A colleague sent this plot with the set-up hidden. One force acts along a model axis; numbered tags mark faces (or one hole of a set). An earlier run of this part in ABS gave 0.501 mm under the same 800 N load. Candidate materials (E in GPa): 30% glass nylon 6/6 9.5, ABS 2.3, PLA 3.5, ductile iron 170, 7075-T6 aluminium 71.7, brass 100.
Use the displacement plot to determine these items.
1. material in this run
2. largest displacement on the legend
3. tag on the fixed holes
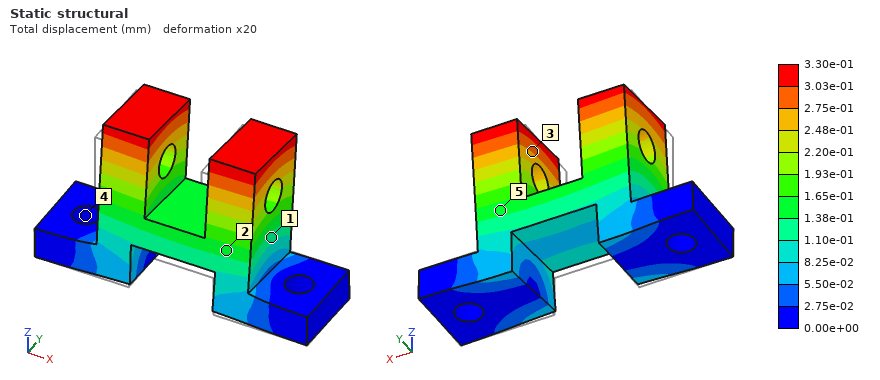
PLA
3.30e-01 mm
4
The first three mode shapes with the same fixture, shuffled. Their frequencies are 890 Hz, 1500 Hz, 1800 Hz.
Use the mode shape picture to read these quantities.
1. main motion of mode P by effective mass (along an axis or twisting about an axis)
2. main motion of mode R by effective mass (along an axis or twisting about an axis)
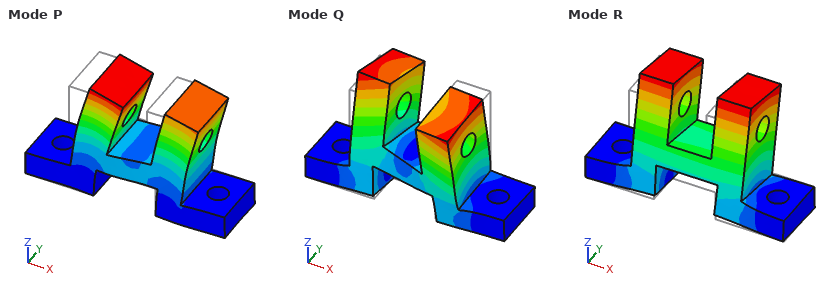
along X
along Y
